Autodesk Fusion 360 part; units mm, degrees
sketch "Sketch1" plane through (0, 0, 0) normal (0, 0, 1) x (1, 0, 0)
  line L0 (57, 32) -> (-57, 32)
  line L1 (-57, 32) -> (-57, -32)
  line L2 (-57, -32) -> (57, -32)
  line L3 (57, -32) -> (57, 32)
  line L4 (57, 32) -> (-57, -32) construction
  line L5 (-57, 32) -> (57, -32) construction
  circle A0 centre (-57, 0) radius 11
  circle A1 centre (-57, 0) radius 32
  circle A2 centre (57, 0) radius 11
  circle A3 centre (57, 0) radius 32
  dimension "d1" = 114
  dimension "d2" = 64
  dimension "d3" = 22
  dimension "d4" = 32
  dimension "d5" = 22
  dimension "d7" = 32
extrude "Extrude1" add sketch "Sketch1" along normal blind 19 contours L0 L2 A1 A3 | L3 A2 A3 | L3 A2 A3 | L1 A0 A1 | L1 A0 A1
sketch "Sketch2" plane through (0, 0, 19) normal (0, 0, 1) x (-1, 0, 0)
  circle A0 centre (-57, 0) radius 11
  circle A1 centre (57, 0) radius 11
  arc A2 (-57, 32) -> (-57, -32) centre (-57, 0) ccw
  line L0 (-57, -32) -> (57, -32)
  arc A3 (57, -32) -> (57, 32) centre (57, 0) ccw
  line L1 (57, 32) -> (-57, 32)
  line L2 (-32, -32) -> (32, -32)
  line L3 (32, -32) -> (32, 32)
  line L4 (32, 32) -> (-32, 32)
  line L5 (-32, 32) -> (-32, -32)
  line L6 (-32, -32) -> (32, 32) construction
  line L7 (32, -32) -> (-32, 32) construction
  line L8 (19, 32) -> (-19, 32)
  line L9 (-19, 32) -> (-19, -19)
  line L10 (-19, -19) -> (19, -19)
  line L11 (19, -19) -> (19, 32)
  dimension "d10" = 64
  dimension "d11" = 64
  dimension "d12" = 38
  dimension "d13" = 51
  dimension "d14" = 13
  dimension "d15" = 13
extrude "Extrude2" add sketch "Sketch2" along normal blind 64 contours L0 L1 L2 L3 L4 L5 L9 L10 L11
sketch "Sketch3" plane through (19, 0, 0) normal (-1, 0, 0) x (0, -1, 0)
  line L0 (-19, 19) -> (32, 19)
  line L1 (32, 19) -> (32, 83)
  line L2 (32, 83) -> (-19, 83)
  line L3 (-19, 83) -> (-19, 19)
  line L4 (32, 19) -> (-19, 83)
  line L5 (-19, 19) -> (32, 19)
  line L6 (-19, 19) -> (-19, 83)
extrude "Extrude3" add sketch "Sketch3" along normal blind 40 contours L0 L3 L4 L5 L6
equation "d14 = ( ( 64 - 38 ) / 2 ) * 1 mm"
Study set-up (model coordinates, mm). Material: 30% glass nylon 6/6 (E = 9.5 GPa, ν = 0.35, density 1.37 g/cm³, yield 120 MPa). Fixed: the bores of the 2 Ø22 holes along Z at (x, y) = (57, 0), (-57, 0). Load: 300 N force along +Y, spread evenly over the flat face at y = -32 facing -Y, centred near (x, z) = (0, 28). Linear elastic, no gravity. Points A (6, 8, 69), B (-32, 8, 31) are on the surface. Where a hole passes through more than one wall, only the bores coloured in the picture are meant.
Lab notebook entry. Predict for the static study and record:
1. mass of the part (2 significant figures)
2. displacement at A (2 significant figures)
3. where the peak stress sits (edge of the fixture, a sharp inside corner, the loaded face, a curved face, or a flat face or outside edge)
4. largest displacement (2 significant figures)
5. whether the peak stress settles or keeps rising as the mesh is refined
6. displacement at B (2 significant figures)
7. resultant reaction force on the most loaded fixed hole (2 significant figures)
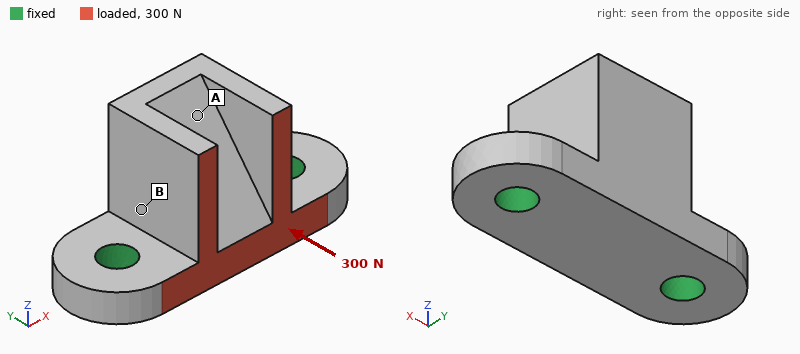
530 g
8.9 µm
edge of the fixture
12 µm
keeps rising
3.9 µm
150 N
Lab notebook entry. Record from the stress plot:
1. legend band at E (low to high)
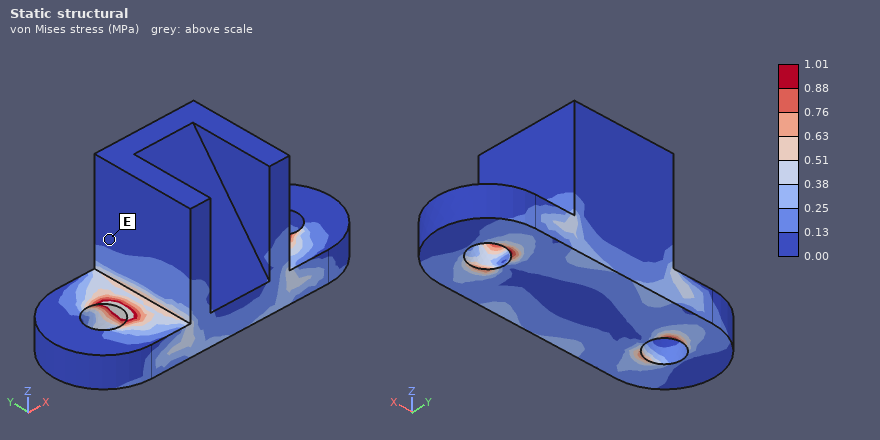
0.00 to 0.13 MPa
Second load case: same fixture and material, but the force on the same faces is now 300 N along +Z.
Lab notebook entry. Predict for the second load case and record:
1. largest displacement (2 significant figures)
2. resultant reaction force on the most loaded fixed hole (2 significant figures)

16 µm
160 N
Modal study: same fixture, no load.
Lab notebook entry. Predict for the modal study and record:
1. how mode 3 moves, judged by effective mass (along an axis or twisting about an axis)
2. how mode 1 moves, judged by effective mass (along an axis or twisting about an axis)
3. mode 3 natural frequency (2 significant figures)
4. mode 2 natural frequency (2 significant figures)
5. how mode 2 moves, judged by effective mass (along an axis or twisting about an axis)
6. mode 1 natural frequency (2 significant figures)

along Z
along Y
2900 Hz
2500 Hz
along X
1300 Hz
